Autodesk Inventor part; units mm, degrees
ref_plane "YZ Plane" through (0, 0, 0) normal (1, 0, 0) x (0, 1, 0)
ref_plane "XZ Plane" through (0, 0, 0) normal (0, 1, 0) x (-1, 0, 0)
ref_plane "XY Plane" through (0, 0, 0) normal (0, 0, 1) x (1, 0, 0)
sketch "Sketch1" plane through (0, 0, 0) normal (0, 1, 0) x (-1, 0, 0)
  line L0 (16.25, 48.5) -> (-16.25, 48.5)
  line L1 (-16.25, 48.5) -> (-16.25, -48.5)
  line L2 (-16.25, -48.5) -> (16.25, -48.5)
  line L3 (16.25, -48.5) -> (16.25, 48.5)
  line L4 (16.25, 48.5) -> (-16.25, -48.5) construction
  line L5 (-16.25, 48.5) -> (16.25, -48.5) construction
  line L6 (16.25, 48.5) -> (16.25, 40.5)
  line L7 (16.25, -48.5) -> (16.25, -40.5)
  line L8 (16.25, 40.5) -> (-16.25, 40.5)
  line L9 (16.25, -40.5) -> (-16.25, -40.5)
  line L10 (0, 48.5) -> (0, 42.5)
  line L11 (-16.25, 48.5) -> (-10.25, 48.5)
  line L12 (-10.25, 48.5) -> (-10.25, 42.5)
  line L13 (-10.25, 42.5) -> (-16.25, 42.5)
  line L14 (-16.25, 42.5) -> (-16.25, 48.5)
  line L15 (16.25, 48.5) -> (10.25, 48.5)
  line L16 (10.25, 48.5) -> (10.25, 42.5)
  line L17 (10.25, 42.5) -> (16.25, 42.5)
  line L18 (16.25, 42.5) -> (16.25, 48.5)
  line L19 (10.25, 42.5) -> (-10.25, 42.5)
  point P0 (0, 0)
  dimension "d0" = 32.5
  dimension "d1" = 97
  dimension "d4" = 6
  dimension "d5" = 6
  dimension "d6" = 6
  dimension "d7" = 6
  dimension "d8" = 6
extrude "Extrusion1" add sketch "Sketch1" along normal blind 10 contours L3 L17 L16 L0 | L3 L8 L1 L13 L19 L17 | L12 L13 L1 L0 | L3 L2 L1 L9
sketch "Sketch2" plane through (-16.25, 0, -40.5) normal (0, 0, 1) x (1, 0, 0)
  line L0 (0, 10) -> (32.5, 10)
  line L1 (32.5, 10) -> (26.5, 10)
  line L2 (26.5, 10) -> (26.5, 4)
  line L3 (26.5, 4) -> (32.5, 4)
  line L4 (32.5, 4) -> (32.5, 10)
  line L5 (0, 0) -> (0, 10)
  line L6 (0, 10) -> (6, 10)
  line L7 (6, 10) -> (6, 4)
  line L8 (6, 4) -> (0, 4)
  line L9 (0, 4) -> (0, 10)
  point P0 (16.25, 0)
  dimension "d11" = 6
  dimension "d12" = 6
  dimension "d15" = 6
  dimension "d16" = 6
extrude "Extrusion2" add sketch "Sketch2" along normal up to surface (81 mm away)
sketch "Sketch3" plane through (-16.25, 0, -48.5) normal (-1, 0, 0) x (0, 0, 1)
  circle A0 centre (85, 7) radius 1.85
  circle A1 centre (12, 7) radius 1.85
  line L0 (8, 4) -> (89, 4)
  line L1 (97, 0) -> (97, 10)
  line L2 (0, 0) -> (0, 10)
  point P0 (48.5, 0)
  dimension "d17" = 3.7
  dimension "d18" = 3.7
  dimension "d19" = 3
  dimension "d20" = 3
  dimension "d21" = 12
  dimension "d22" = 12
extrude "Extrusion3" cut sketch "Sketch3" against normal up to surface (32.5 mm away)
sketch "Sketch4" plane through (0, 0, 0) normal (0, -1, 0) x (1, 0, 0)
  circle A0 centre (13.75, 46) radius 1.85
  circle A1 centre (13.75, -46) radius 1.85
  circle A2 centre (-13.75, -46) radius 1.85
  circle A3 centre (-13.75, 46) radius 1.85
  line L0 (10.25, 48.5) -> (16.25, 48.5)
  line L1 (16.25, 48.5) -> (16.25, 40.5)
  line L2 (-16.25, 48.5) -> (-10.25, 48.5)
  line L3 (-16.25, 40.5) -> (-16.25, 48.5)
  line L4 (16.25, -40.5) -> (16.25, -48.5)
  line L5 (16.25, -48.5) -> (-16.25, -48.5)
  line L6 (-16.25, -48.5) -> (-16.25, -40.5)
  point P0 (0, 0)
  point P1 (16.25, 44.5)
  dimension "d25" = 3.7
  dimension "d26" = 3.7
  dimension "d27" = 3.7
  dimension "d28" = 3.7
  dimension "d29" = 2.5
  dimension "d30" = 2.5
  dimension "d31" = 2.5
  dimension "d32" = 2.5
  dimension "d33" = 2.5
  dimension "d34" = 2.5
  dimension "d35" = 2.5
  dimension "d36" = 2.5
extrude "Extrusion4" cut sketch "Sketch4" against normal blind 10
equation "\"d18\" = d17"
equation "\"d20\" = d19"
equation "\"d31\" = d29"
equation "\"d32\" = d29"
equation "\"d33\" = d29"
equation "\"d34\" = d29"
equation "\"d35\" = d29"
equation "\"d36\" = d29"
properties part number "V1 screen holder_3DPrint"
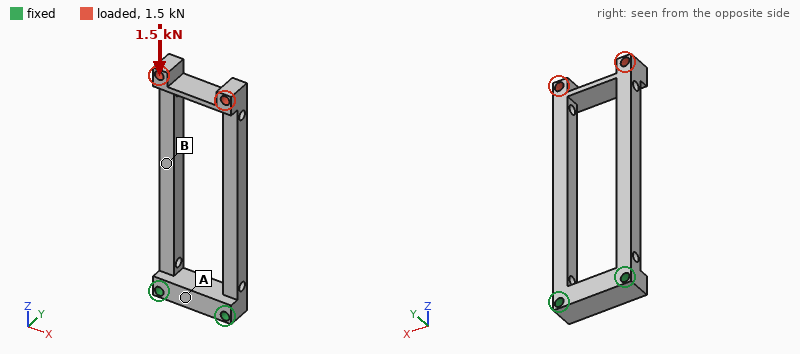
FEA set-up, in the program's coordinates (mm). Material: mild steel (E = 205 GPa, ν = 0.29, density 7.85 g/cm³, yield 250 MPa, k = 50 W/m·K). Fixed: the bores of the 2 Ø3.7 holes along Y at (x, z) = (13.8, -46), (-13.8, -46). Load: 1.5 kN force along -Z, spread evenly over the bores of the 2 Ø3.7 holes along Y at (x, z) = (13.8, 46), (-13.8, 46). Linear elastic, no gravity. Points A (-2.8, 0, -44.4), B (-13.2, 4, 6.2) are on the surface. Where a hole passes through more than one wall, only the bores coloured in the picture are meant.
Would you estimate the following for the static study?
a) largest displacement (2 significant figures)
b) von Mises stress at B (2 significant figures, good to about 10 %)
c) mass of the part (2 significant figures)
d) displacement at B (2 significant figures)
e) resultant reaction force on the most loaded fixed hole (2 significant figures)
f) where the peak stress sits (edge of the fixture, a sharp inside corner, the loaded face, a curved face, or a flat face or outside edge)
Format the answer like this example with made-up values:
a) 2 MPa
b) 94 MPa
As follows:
a) 0.29 mm
b) 63 MPa
c) 72 g
d) 0.084 mm
e) 750 N
f) a curved face
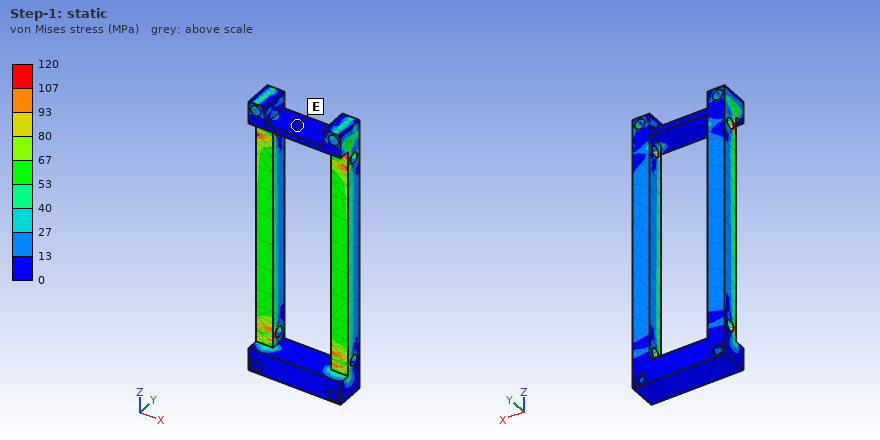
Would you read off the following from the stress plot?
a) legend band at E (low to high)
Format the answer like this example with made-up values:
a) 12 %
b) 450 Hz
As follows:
a) 0 to 13 MPa
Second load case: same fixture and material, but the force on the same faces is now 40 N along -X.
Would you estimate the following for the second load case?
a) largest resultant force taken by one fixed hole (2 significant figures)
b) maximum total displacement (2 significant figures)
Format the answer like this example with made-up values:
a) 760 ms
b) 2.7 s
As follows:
a) 96 N
b) 0.13 mm
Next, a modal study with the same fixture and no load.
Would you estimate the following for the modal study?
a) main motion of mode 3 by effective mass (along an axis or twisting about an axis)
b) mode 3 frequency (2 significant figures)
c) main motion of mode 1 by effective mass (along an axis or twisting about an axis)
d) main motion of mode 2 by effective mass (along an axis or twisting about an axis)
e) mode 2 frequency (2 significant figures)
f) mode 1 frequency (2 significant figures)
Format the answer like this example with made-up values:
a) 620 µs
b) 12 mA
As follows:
a) twisting about Z
b) 1600 Hz
c) along Y
d) along X
e) 640 Hz
f) 520 Hz
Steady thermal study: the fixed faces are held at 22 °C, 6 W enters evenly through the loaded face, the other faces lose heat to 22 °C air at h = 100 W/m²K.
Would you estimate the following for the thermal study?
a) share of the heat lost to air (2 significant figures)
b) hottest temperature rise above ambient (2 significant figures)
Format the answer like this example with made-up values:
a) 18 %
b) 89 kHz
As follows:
a) 96 %
b) 33 K
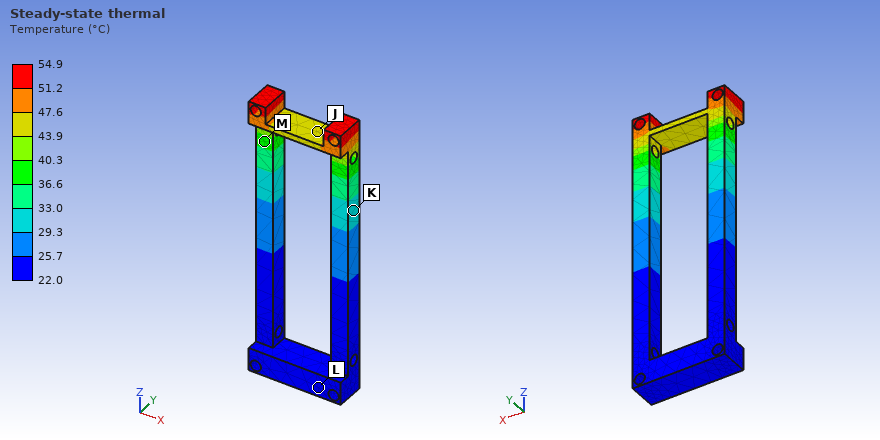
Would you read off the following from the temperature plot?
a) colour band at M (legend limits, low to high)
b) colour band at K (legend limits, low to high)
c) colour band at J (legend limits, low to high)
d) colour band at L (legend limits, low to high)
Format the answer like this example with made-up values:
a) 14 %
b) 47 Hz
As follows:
a) 36.6 to 40.3 °C
b) 29.3 to 33.0 °C
c) 43.9 to 47.6 °C
d) 22.0 to 25.7 °C
